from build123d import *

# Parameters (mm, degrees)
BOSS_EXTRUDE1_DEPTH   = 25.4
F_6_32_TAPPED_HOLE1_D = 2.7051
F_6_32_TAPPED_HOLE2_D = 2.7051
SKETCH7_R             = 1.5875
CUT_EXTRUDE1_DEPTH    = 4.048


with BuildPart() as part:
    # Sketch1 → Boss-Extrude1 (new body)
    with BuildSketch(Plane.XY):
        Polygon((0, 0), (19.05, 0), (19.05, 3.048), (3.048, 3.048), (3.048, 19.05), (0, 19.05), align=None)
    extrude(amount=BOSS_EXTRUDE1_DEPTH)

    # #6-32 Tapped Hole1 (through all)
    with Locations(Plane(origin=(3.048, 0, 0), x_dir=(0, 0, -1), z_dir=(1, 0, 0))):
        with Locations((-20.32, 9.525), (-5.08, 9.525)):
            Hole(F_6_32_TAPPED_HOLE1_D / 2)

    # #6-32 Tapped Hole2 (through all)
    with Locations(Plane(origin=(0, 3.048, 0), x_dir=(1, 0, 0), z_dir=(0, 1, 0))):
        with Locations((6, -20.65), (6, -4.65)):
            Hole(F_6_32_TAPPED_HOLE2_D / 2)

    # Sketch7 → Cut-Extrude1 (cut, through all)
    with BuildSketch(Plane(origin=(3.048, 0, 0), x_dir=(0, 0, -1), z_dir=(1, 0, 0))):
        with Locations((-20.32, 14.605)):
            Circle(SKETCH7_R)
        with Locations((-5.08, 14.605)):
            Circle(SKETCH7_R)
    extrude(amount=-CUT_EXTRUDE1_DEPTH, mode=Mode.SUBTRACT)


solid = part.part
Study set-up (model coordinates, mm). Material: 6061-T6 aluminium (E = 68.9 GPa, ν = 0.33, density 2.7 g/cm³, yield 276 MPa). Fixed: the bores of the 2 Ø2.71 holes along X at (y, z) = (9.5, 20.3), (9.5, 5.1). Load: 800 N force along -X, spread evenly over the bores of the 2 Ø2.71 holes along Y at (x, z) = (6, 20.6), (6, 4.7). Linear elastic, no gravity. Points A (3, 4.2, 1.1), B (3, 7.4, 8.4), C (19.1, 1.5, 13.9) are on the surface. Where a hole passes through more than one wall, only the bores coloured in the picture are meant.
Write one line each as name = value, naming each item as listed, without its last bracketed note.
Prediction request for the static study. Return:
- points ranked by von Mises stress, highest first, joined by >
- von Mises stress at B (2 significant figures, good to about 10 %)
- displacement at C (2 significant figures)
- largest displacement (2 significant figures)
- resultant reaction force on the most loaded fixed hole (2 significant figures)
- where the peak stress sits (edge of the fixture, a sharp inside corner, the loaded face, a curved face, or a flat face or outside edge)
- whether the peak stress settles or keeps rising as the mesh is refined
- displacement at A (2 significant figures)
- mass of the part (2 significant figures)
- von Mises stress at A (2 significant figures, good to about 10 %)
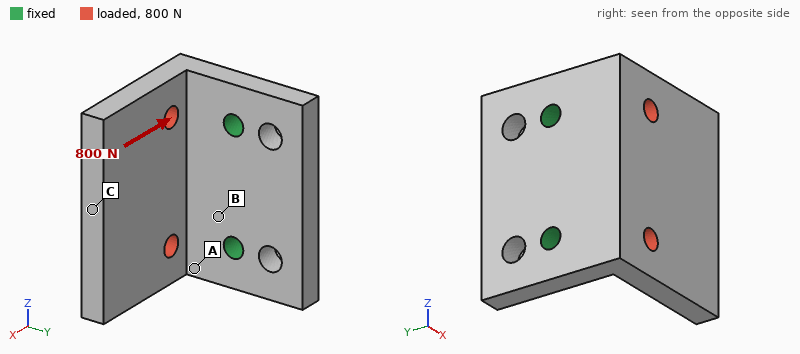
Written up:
points ranked by von Mises stress, highest first, joined by > = B > A > C
von Mises stress at B = 82 MPa
displacement at C = 0.12 mm
largest displacement = 0.12 mm
resultant reaction force on the most loaded fixed hole = 400 N
where the peak stress sits = edge of the fixture
whether the peak stress settles or keeps rising as the mesh is refined = keeps rising
displacement at A = 0.022 mm
mass of the part = 7.0 g
von Mises stress at A = 52 MPa
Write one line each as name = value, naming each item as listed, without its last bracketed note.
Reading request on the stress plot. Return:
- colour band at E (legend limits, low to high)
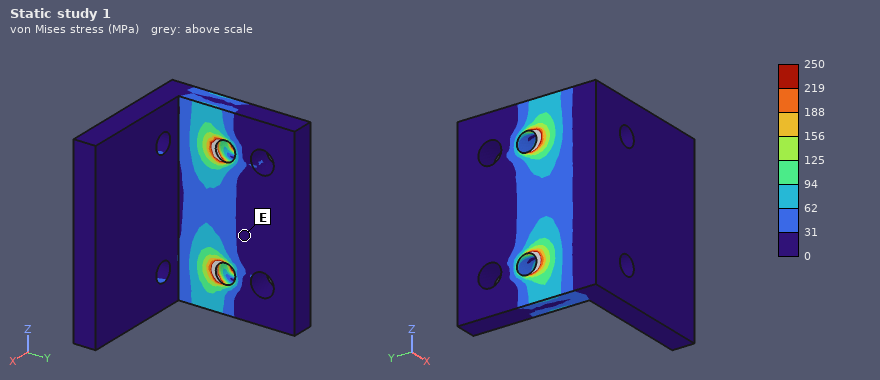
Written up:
colour band at E = 0 to 31 MPa
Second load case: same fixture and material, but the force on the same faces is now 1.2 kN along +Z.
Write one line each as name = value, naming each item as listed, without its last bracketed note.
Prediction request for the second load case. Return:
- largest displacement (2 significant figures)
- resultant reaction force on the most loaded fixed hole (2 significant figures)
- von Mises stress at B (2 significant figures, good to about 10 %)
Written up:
largest displacement = 51 µm
resultant reaction force on the most loaded fixed hole = 860 N
von Mises stress at B = 62 MPa
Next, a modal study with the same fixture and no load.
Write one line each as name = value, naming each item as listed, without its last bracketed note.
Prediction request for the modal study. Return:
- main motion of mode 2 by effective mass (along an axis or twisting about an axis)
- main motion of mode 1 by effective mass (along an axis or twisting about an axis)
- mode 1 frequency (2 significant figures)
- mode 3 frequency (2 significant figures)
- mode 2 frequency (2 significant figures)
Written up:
main motion of mode 2 by effective mass = along Z
main motion of mode 1 by effective mass = along Y
mode 1 frequency = 4800 Hz
mode 3 frequency = 14 kHz
mode 2 frequency = 9500 Hz
